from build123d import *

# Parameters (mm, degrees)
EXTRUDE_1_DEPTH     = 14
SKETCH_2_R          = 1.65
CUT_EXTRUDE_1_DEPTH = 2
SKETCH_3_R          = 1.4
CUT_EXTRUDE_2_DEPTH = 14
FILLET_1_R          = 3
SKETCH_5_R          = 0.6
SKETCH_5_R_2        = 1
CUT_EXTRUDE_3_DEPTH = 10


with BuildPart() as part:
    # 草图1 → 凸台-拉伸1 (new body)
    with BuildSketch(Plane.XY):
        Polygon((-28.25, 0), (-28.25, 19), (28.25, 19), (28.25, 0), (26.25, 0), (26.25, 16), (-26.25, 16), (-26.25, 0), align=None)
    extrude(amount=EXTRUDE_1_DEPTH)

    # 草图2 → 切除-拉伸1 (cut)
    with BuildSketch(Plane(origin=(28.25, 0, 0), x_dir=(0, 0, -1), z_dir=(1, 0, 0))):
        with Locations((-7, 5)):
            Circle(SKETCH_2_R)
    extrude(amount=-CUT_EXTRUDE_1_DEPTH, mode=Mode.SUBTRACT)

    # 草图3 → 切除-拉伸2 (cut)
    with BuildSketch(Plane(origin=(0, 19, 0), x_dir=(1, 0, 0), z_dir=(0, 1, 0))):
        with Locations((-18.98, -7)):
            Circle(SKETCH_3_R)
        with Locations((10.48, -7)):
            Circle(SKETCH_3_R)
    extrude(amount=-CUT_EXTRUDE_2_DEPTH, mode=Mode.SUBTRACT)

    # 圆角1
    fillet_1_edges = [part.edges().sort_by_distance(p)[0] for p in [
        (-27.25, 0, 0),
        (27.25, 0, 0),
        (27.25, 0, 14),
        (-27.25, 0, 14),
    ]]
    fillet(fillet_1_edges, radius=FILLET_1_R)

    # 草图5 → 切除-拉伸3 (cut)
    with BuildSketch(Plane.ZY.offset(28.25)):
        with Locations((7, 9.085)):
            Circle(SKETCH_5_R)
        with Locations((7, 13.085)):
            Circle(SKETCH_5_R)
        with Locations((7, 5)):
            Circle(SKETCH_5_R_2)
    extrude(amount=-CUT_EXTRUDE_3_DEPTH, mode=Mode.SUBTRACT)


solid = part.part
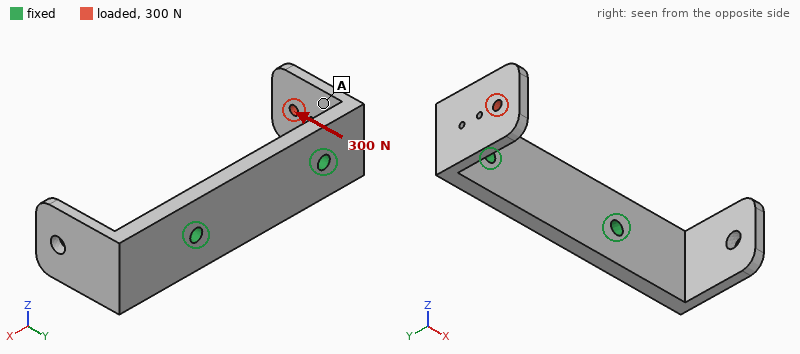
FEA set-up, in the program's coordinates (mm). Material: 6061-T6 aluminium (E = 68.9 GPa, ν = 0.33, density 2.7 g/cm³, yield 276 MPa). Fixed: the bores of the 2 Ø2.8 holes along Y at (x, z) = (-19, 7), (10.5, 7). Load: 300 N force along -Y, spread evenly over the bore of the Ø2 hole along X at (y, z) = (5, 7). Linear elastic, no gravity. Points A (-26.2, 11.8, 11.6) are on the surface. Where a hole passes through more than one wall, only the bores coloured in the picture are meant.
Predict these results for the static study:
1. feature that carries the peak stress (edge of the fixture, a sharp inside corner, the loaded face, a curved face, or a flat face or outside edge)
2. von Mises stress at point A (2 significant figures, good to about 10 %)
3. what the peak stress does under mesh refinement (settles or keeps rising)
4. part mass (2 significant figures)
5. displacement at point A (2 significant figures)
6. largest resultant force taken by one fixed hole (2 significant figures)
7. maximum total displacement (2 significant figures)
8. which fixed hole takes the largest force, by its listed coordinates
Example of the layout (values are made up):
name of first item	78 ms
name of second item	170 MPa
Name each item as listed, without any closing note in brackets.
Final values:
feature that carries the peak stress	edge of the fixture
von Mises stress at point A	10 MPa
what the peak stress does under mesh refinement	keeps rising
part mass	8.6 g
displacement at point A	37 µm
largest resultant force taken by one fixed hole	310 N
maximum total displacement	92 µm
which fixed hole takes the largest force, by its listed coordinates	(-19, 7)
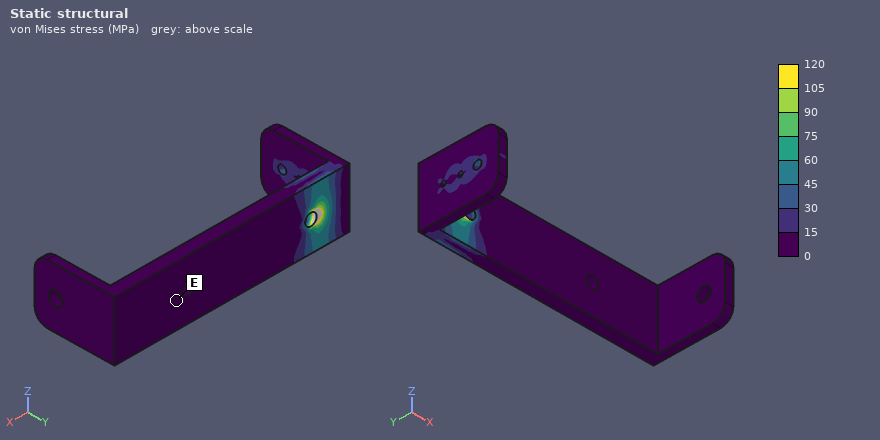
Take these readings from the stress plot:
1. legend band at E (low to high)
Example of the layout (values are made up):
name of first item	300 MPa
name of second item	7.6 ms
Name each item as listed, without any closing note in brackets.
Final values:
legend band at E	0 to 15 MPa
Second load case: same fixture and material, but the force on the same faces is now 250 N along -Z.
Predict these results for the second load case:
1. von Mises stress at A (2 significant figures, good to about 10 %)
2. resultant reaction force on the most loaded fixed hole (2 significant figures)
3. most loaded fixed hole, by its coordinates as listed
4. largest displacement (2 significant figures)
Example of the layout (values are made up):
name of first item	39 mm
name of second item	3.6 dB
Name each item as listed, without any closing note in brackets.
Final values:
von Mises stress at A	45 MPa
resultant reaction force on the most loaded fixed hole	300 N
most loaded fixed hole, by its coordinates as listed	(-19, 7)
largest displacement	0.16 mm
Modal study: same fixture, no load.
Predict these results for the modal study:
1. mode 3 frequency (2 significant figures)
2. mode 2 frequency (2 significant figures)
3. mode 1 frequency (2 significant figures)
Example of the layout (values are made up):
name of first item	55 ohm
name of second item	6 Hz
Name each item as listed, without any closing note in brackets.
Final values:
mode 3 frequency	5200 Hz
mode 2 frequency	4600 Hz
mode 1 frequency	3300 Hz
